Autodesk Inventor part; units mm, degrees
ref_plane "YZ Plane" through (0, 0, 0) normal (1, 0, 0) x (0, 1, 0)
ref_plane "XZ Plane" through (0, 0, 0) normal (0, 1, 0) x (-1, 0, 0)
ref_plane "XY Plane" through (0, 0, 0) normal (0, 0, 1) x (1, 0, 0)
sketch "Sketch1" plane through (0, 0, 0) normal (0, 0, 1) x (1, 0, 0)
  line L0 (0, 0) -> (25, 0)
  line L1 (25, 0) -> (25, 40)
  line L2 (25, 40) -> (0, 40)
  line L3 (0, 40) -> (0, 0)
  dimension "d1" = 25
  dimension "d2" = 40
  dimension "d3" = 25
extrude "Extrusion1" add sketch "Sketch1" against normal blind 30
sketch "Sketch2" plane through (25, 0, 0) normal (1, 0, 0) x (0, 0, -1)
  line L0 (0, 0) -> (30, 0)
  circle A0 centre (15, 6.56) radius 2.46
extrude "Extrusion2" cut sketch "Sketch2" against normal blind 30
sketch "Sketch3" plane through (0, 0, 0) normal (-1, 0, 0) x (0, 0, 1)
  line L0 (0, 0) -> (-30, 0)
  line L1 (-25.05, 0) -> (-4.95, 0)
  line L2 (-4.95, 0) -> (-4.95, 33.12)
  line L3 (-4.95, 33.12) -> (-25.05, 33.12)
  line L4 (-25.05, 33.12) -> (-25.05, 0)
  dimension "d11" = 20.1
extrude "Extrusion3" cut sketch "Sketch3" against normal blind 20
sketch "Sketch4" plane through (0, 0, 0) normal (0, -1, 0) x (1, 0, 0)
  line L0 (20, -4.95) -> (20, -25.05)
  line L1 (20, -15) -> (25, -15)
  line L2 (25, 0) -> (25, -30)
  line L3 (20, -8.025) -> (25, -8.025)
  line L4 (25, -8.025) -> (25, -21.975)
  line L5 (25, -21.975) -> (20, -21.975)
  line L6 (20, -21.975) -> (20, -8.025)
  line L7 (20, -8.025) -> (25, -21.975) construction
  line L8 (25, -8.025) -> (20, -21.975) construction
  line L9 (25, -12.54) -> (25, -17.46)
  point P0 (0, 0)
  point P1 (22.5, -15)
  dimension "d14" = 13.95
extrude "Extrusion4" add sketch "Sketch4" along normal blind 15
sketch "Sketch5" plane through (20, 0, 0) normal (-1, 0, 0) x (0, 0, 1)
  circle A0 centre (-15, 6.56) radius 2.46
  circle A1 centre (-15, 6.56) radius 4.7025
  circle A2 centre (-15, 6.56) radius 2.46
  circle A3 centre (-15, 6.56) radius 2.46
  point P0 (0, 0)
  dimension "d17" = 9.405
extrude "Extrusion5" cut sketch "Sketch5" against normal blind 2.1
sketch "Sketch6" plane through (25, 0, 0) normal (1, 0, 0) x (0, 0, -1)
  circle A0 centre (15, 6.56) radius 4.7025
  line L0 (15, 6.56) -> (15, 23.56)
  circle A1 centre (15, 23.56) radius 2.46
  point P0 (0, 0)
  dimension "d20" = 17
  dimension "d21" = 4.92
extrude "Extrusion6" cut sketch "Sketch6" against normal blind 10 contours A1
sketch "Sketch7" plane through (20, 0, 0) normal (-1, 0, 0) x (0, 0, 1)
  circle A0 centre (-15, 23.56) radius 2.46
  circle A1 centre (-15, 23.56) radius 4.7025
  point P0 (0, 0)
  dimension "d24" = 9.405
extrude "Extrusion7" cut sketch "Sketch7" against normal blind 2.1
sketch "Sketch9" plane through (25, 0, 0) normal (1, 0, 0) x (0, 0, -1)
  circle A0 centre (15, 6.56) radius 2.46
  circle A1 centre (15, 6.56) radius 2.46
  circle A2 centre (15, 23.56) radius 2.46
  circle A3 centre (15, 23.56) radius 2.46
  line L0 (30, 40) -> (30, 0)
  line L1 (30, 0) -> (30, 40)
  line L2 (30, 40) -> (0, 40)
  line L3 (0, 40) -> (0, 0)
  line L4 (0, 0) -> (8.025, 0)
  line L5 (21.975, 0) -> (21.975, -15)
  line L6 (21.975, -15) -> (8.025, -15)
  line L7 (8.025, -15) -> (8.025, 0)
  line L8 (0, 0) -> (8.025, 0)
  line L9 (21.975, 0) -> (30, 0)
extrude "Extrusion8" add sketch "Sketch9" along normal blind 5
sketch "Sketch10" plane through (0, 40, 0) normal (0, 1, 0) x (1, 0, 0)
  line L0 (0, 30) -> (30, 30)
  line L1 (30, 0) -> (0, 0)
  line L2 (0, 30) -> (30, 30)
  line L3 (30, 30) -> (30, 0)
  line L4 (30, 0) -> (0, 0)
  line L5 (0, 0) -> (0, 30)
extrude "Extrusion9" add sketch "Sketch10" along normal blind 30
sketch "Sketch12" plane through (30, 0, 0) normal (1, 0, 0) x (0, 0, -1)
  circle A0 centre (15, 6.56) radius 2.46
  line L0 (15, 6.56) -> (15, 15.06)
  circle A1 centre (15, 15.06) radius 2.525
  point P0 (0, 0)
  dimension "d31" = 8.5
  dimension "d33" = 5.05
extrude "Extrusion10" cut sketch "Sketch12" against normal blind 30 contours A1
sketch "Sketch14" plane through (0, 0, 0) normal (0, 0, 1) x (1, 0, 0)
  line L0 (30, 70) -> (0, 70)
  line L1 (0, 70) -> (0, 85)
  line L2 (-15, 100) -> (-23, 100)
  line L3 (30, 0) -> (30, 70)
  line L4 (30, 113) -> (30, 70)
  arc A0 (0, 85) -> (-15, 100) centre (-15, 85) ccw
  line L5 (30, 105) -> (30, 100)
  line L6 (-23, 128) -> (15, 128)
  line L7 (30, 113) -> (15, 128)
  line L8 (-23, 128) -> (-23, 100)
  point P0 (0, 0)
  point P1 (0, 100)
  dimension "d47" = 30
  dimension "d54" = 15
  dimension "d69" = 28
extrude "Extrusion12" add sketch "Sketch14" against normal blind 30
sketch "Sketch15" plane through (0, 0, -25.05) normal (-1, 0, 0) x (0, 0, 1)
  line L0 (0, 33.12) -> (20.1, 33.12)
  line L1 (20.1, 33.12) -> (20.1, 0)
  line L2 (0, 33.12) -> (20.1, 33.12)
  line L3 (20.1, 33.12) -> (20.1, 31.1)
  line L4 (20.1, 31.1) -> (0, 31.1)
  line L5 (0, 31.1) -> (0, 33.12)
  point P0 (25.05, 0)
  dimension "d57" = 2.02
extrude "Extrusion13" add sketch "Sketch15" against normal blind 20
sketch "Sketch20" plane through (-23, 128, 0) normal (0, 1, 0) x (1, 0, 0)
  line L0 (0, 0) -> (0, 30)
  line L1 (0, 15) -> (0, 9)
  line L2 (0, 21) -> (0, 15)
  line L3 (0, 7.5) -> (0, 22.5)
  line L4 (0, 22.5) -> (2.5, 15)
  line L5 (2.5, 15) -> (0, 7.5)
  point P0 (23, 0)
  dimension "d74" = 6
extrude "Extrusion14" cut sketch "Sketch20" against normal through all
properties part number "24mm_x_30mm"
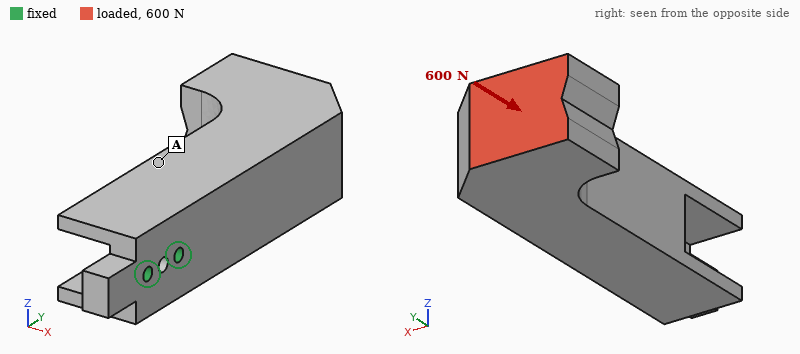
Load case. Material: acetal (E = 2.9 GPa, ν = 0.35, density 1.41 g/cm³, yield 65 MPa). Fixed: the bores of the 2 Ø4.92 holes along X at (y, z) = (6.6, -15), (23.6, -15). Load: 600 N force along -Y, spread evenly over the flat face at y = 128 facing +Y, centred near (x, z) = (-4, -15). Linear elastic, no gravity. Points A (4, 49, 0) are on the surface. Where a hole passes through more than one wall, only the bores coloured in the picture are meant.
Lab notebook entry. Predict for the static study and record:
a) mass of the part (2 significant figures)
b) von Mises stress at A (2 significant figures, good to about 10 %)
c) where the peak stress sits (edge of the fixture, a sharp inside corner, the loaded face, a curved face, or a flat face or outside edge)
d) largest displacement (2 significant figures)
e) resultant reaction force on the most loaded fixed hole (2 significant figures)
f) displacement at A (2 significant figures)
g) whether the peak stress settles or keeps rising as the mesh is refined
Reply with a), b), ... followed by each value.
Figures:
a) 170 g
b) 3.0 MPa
c) edge of the fixture
d) 1.4 mm
e) 800 N
f) 0.33 mm
g) keeps rising
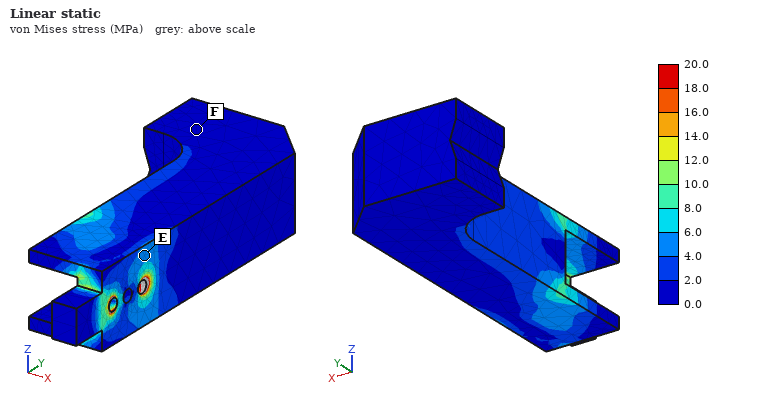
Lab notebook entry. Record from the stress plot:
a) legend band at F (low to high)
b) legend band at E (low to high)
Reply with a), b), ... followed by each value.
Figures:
a) 0.0 to 2.0 MPa
b) 4.0 to 6.0 MPa
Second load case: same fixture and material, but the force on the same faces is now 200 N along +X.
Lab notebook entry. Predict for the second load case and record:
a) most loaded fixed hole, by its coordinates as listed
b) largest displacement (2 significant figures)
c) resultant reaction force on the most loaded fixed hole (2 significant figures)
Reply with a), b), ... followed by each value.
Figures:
a) (23.6, -15)
b) 1.7 mm
c) 1.0 kN
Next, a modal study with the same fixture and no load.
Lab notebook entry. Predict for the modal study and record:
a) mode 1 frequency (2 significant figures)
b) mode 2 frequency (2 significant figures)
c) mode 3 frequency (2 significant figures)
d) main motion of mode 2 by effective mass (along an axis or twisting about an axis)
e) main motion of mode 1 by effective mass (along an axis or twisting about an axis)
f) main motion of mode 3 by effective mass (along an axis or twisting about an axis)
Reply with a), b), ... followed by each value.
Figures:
a) 230 Hz
b) 270 Hz
c) 730 Hz
d) along Z
e) along X
f) twisting about Y
